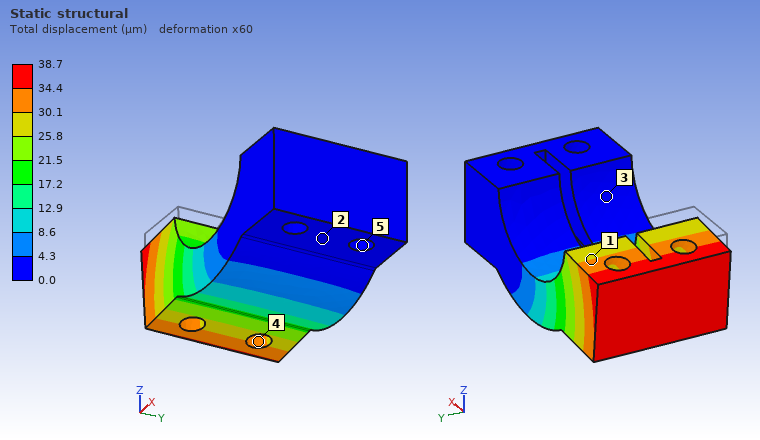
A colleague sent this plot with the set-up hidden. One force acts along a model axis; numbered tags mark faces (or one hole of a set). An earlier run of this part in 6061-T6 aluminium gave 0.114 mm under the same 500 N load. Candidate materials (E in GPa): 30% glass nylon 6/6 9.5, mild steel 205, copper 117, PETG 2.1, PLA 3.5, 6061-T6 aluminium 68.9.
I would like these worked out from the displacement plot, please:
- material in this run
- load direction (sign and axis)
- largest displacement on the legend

mild steel
-Z
38.7 µm
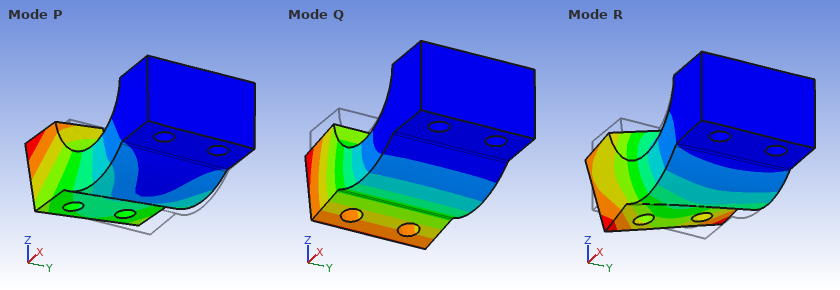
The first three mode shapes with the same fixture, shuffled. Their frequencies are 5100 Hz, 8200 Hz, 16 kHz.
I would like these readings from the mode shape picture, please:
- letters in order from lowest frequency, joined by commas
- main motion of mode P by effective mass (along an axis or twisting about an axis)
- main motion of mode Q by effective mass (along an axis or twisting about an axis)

Q, P, R
along Y
along Z
